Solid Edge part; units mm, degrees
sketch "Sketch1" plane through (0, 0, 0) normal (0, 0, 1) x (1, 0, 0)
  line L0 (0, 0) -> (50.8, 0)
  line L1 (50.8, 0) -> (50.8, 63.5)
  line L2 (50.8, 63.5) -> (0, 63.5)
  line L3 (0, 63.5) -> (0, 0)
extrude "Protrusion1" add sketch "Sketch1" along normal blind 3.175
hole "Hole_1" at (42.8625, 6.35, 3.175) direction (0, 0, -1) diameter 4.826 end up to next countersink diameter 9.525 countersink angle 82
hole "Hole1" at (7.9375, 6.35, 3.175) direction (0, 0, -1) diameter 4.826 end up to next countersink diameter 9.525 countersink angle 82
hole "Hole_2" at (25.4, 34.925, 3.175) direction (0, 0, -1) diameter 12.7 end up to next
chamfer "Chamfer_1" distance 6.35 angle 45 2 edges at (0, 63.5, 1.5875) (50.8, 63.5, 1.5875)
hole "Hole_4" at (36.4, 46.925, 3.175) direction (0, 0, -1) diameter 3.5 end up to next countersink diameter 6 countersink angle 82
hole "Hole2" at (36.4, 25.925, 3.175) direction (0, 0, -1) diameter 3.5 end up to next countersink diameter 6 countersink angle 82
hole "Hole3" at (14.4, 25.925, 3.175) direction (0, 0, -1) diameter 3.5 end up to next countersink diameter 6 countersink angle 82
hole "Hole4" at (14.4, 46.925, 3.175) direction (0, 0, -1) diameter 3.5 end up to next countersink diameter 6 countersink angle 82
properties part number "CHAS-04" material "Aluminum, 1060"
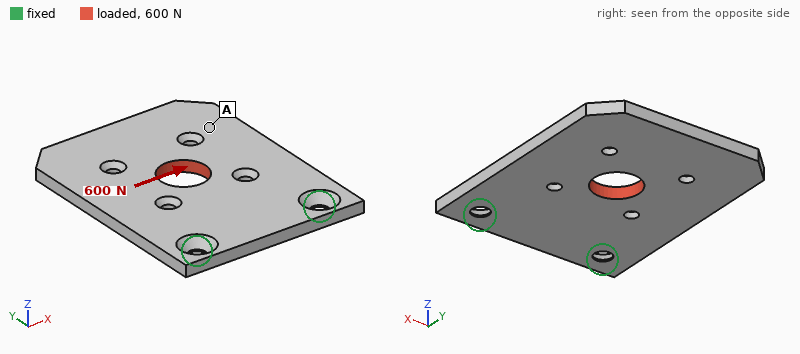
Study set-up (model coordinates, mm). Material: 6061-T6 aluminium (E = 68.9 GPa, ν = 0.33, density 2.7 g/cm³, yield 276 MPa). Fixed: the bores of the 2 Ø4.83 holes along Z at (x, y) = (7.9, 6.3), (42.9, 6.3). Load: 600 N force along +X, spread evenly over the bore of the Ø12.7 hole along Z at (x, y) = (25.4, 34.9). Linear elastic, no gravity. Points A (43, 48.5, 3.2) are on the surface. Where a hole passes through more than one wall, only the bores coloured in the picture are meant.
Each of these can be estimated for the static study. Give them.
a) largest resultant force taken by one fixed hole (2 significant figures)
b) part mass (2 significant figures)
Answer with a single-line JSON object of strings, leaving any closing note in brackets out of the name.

{"largest resultant force taken by one fixed hole": "550 N", "part mass": "25 g"}
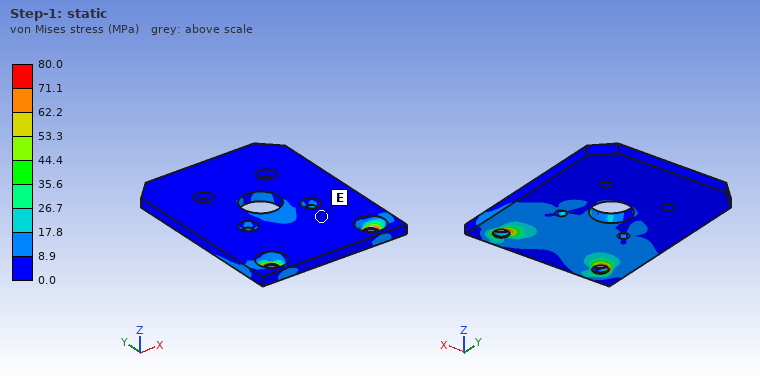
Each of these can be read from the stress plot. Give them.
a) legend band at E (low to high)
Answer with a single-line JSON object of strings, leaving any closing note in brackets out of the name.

{"legend band at E": "0.0 to 8.9 MPa"}
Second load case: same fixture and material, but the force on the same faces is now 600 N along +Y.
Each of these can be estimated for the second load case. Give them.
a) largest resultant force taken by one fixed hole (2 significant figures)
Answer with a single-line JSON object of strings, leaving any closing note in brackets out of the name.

{"largest resultant force taken by one fixed hole": "300 N"}
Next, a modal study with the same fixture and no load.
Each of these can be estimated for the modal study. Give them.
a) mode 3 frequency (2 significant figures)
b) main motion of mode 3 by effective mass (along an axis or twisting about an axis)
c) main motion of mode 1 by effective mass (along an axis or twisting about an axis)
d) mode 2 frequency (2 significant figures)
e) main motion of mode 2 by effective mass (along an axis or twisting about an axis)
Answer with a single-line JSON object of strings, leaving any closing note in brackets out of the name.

{"mode 3 frequency": "3800 Hz", "main motion of mode 3 by effective mass": "along Z", "main motion of mode 1 by effective mass": "along Z", "mode 2 frequency": "1900 Hz", "main motion of mode 2 by effective mass": "twisting about Y"}
